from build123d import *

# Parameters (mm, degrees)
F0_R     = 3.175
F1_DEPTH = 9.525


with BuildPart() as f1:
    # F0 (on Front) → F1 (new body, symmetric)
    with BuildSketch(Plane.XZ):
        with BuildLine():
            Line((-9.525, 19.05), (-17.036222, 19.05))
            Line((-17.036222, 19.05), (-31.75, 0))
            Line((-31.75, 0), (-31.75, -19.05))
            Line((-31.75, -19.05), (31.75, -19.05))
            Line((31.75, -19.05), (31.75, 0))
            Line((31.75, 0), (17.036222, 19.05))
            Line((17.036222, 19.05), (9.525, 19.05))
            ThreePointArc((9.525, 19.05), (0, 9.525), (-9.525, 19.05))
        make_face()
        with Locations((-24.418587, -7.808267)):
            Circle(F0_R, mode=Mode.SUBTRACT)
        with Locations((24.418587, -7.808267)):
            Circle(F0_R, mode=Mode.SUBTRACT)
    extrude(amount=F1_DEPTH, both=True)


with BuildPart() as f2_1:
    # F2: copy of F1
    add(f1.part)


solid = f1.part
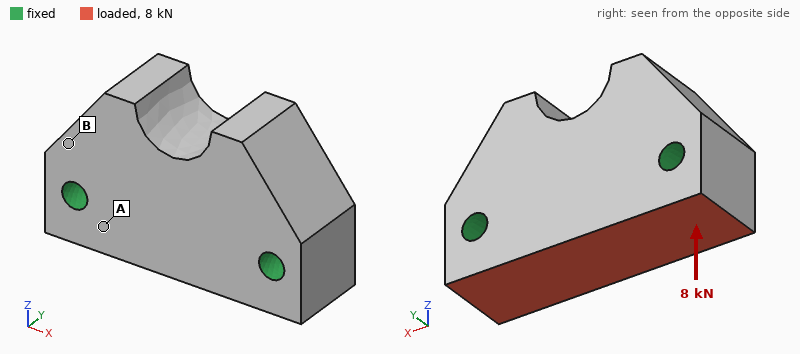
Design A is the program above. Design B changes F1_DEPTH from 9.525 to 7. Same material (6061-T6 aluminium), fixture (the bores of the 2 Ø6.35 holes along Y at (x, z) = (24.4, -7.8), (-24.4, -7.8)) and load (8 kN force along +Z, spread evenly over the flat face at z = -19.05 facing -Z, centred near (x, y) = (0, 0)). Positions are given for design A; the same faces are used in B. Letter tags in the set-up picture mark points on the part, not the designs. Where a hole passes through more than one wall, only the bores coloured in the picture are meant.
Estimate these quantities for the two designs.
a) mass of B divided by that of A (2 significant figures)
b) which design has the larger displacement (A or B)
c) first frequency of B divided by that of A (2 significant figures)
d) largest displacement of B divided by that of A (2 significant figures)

0.73
B
0.84
1.3
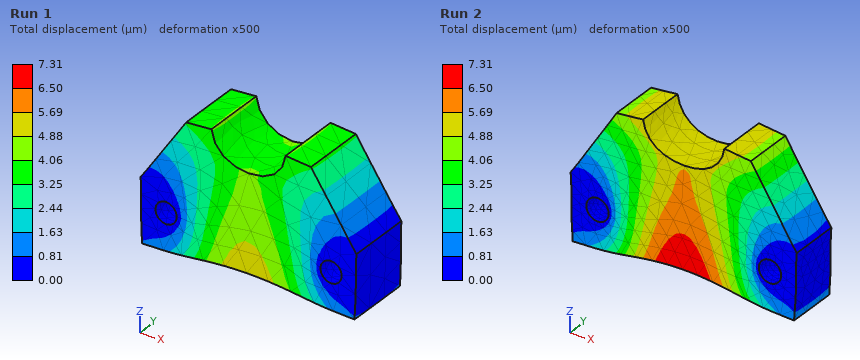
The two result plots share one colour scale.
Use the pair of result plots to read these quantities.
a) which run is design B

Run 2
